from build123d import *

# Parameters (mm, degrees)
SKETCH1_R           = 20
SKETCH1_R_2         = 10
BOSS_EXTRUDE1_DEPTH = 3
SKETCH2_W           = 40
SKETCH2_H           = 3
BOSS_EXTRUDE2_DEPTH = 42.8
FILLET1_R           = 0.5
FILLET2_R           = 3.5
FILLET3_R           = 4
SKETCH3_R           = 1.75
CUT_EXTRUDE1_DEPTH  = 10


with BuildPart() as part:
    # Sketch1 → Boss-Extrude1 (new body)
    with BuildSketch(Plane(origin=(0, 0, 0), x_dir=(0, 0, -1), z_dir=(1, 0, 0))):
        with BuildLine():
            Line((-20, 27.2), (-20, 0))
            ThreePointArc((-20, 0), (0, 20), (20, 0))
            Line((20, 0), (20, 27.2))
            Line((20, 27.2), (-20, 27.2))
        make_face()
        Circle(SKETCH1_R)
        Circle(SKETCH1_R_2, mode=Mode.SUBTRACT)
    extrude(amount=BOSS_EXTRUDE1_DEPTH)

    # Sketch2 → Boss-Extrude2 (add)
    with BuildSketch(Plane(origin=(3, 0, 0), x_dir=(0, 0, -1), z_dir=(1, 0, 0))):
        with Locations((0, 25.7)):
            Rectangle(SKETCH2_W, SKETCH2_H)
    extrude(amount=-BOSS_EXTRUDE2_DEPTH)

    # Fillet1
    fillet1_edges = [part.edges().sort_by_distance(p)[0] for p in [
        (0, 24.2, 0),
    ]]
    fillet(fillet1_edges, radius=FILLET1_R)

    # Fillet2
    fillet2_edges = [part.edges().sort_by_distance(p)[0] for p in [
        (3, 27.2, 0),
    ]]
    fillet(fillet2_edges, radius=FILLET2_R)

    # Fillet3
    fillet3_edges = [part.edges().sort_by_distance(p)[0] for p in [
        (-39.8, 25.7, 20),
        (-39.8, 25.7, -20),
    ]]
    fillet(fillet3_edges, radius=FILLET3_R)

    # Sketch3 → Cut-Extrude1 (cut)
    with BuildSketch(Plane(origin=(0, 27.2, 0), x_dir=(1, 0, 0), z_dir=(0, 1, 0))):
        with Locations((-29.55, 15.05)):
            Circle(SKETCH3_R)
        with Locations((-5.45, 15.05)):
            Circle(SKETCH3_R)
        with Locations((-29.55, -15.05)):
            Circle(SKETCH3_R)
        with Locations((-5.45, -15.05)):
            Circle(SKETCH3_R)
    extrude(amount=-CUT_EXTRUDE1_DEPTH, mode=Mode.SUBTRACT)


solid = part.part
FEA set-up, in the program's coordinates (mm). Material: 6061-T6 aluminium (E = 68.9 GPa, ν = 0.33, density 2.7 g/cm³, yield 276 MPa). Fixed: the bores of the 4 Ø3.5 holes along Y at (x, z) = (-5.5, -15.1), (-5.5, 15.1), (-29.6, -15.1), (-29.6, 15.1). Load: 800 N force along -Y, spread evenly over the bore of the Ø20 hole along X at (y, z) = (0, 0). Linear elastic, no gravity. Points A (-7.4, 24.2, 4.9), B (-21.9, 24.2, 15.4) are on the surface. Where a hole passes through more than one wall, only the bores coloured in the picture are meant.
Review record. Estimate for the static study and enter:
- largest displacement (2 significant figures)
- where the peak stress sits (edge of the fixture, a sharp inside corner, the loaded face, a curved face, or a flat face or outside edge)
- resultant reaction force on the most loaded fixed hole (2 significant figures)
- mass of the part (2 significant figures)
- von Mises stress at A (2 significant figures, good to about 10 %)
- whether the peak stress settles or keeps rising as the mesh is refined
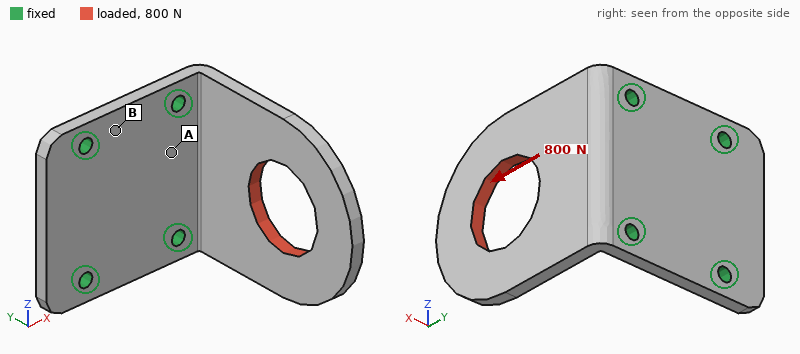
0.15 mm
edge of the fixture
420 N
24 g
21 MPa
keeps rising
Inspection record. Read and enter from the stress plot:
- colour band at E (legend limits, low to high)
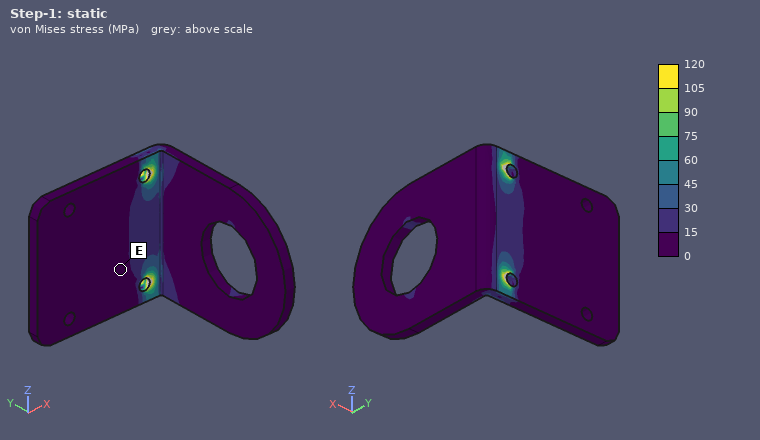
0 to 15 MPa
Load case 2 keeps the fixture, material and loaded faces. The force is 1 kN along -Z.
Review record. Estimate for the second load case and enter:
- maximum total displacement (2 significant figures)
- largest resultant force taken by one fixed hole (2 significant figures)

0.14 mm
990 N
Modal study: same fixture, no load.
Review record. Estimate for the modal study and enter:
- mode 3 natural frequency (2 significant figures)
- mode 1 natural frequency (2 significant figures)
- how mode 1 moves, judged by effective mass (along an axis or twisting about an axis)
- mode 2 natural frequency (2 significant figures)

5900 Hz
1200 Hz
along X
3300 Hz
